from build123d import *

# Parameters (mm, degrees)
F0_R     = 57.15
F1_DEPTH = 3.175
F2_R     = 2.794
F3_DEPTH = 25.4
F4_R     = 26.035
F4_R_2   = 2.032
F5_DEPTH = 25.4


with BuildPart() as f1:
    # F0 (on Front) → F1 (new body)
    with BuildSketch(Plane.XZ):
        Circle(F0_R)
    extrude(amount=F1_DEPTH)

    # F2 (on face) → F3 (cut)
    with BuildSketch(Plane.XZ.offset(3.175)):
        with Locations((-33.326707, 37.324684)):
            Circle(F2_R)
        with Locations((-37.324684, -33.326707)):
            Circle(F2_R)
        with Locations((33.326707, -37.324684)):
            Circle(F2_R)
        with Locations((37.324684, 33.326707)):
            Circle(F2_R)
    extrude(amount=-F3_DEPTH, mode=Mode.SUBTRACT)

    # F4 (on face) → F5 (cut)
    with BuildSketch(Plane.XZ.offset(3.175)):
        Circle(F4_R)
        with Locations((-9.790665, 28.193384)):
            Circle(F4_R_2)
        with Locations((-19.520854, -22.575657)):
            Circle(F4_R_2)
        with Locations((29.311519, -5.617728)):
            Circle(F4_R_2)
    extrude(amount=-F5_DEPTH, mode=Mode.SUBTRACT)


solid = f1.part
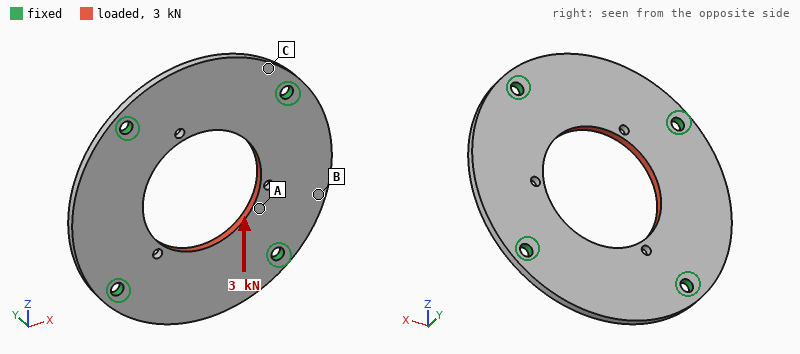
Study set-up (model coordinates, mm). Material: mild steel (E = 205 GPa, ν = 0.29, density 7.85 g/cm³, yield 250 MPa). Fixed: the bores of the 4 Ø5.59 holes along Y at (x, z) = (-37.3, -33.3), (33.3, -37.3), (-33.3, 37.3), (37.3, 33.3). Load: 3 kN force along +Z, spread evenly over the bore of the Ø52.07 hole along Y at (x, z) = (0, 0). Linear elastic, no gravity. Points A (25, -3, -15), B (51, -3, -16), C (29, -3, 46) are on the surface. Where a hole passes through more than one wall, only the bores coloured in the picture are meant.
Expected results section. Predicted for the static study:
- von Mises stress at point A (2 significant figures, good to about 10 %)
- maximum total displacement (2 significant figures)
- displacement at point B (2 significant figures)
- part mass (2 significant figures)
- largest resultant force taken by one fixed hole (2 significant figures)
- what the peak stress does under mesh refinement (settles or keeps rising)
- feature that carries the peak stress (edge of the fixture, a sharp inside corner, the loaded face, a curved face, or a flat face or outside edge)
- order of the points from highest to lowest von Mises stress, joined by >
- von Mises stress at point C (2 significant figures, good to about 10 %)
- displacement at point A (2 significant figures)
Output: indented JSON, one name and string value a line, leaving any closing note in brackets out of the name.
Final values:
{
  "von Mises stress at point A": "11 MPa",
  "maximum total displacement": "2.6 µm",
  "displacement at point B": "0.60 µm",
  "part mass": "200 g",
  "largest resultant force taken by one fixed hole": "760 N",
  "what the peak stress does under mesh refinement": "keeps rising",
  "feature that carries the peak stress": "edge of the fixture",
  "order of the points from highest to lowest von Mises stress, joined by >": "A > C > B",
  "von Mises stress at point C": "5.6 MPa",
  "displacement at point A": "1.2 µm"
}
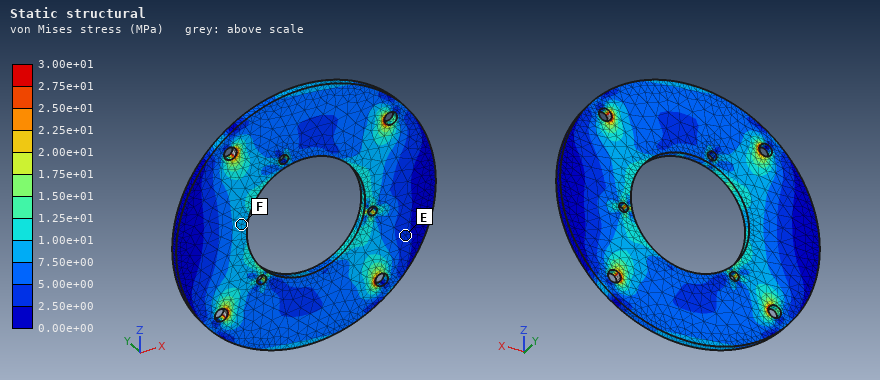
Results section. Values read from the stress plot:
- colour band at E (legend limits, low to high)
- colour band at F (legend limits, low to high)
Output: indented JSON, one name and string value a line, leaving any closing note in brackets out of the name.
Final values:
{
  "colour band at E": "2.50e+00 to 5.00e+00 MPa",
  "colour band at F": "7.50e+00 to 1.00e+01 MPa"
}
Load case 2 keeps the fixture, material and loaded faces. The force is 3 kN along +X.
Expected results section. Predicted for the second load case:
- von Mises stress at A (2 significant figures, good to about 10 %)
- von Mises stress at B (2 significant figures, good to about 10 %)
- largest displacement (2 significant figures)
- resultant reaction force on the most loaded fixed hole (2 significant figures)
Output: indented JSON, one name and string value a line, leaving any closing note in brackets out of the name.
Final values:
{
  "von Mises stress at A": "4.9 MPa",
  "von Mises stress at B": "6.9 MPa",
  "largest displacement": "2.7 µm",
  "resultant reaction force on the most loaded fixed hole": "760 N"
}
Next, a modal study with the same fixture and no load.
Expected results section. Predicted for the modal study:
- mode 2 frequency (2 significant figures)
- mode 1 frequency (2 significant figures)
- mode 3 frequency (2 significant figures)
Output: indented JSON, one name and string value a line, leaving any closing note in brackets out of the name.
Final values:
{
  "mode 2 frequency": "2900 Hz",
  "mode 1 frequency": "2700 Hz",
  "mode 3 frequency": "2900 Hz"
}
